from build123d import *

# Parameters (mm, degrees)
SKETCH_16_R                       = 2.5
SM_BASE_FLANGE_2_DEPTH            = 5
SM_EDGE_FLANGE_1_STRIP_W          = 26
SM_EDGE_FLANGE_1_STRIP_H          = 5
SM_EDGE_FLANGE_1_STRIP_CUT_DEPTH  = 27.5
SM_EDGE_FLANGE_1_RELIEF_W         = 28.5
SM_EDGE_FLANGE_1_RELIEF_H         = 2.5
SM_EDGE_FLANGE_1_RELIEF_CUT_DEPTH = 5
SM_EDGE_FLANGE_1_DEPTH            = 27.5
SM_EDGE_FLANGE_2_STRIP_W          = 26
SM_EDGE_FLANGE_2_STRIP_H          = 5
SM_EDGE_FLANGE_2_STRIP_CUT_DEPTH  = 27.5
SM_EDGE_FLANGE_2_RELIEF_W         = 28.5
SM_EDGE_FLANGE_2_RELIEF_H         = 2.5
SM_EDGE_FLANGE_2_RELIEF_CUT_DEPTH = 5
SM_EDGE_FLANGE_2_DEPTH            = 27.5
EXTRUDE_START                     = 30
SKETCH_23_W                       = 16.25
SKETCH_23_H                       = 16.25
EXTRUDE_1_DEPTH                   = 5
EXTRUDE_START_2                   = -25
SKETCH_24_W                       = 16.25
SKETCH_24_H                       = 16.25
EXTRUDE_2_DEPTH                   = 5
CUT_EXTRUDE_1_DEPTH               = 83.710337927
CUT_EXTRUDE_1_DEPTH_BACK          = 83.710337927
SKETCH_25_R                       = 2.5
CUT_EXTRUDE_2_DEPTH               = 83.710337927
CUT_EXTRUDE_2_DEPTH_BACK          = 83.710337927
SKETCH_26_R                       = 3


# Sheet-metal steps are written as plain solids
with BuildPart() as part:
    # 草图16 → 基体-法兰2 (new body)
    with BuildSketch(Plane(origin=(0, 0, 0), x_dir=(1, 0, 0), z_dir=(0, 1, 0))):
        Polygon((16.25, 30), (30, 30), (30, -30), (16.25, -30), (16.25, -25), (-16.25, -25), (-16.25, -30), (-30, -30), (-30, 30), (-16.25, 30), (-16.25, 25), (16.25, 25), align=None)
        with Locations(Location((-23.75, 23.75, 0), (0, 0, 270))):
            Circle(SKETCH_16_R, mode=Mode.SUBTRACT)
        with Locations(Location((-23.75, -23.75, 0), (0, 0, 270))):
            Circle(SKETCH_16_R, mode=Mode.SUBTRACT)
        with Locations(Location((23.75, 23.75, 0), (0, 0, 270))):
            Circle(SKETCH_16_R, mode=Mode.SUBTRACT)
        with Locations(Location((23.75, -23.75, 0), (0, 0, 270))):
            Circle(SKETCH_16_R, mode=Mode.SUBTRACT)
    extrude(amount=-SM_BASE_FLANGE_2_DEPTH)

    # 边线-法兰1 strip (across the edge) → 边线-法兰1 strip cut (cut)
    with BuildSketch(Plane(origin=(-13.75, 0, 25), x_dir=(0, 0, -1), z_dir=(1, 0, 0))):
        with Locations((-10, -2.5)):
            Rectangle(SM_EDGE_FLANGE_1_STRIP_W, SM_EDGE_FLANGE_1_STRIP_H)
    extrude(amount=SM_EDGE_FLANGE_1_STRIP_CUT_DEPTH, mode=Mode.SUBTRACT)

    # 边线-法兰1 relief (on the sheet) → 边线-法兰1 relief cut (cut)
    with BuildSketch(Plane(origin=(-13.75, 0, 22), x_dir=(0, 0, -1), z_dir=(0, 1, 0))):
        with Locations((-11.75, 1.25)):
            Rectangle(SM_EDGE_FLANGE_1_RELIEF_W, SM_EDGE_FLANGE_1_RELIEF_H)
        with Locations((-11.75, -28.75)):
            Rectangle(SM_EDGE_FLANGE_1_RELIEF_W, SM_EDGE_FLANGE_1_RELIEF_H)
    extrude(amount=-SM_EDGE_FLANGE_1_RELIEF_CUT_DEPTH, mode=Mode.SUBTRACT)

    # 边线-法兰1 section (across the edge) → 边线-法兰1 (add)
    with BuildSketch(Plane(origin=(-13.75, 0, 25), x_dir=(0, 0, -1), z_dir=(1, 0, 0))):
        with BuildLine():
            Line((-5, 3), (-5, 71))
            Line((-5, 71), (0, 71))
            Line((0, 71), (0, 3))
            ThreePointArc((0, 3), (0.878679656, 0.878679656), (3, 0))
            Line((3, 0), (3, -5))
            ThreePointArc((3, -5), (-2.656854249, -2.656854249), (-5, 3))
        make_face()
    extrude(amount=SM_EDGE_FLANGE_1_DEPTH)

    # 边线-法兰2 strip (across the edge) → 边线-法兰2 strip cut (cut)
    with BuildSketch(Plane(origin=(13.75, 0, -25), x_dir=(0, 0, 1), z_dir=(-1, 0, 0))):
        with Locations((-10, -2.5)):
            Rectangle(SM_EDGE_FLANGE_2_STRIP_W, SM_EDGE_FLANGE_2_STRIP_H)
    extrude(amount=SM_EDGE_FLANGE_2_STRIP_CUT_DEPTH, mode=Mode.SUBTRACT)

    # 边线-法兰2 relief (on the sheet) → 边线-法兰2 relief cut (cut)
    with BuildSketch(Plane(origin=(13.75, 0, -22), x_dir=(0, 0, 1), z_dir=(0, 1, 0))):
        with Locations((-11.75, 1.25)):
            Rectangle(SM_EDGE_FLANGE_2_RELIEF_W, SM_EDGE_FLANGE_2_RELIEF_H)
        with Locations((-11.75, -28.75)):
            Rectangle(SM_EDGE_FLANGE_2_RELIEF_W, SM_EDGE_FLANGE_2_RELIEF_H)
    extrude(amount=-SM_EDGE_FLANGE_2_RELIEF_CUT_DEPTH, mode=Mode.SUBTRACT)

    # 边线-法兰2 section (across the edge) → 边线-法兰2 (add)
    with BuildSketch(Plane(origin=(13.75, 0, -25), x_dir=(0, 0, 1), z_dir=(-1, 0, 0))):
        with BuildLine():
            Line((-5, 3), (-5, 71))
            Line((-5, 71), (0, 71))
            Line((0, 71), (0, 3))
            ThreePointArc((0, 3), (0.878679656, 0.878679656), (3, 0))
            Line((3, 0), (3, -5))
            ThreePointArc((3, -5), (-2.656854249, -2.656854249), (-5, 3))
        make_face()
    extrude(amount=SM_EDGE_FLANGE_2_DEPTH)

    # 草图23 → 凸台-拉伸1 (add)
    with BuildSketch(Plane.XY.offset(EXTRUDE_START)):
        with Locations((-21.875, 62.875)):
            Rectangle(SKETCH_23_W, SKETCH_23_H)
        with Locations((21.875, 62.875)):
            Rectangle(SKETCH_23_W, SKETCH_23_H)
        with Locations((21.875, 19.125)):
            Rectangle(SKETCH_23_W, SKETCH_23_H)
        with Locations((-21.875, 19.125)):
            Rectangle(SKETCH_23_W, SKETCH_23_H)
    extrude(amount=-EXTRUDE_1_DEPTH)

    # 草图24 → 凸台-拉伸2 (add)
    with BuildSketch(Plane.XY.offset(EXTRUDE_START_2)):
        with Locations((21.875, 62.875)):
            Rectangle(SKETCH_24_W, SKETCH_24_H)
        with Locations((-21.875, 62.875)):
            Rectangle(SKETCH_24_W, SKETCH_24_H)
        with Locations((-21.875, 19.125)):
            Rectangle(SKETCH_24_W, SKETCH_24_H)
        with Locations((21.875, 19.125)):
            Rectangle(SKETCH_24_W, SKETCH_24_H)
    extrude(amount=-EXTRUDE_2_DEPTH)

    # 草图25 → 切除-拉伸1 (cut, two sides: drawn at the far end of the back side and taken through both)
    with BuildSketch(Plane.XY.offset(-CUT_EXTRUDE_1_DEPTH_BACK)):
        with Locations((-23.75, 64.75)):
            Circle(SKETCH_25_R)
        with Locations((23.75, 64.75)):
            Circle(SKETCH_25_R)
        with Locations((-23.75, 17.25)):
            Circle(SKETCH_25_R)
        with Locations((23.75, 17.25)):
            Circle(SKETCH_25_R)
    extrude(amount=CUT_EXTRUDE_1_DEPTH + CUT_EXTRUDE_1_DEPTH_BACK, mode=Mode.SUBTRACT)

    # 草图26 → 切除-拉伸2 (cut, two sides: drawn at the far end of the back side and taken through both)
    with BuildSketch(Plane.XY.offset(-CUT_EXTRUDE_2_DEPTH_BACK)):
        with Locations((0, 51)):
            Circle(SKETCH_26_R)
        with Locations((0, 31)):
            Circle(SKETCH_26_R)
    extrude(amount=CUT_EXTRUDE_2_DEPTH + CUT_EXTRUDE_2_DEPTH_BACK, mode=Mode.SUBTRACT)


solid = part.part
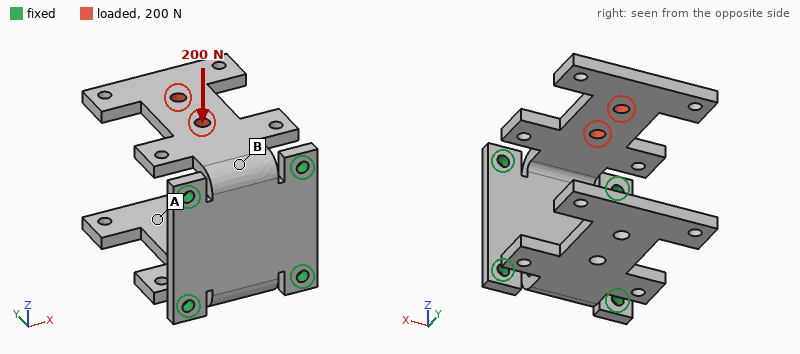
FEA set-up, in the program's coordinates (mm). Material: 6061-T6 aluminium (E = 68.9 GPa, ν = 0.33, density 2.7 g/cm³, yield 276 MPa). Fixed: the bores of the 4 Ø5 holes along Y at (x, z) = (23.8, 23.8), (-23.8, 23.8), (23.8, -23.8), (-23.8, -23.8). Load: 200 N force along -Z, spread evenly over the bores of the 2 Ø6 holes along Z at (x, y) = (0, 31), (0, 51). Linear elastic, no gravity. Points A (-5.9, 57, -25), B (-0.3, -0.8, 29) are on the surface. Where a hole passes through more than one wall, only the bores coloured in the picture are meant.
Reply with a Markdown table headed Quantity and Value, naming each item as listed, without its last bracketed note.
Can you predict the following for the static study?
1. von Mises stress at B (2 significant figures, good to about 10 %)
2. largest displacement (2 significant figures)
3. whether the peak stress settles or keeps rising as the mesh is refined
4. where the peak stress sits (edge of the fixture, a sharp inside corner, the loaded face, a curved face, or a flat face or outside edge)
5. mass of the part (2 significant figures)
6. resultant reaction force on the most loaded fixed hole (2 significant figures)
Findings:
| Quantity | Value |
|---|---|
| von Mises stress at B | 51 MPa |
| largest displacement | 1.00 mm |
| whether the peak stress settles or keeps rising as the mesh is refined | keeps rising |
| where the peak stress sits | a sharp inside corner |
| mass of the part | 120 g |
| resultant reaction force on the most loaded fixed hole | 120 N |
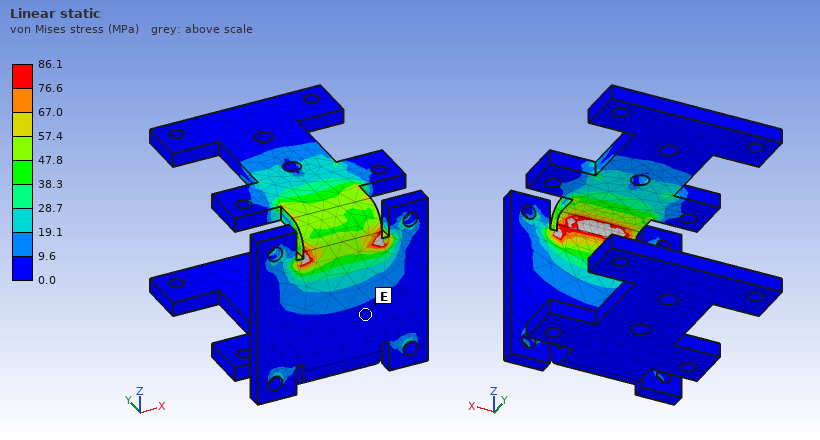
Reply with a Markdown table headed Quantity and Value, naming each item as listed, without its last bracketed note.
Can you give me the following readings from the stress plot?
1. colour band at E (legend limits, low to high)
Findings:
| Quantity | Value |
|---|---|
| colour band at E | 0.0 to 9.6 MPa |
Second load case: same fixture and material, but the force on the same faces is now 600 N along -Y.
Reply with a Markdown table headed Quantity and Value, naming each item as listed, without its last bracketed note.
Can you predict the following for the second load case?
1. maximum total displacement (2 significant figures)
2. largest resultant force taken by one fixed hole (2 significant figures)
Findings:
| Quantity | Value |
|---|---|
| maximum total displacement | 0.32 mm |
| largest resultant force taken by one fixed hole | 360 N |
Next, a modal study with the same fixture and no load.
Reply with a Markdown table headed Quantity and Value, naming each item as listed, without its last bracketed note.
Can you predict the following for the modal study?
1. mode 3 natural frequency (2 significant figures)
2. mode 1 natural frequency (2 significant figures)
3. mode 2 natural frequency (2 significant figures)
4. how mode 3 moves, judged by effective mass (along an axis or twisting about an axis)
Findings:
| Quantity | Value |
|---|---|
| mode 3 natural frequency | 1000 Hz |
| mode 1 natural frequency | 440 Hz |
| mode 2 natural frequency | 450 Hz |
| how mode 3 moves, judged by effective mass | along X |
